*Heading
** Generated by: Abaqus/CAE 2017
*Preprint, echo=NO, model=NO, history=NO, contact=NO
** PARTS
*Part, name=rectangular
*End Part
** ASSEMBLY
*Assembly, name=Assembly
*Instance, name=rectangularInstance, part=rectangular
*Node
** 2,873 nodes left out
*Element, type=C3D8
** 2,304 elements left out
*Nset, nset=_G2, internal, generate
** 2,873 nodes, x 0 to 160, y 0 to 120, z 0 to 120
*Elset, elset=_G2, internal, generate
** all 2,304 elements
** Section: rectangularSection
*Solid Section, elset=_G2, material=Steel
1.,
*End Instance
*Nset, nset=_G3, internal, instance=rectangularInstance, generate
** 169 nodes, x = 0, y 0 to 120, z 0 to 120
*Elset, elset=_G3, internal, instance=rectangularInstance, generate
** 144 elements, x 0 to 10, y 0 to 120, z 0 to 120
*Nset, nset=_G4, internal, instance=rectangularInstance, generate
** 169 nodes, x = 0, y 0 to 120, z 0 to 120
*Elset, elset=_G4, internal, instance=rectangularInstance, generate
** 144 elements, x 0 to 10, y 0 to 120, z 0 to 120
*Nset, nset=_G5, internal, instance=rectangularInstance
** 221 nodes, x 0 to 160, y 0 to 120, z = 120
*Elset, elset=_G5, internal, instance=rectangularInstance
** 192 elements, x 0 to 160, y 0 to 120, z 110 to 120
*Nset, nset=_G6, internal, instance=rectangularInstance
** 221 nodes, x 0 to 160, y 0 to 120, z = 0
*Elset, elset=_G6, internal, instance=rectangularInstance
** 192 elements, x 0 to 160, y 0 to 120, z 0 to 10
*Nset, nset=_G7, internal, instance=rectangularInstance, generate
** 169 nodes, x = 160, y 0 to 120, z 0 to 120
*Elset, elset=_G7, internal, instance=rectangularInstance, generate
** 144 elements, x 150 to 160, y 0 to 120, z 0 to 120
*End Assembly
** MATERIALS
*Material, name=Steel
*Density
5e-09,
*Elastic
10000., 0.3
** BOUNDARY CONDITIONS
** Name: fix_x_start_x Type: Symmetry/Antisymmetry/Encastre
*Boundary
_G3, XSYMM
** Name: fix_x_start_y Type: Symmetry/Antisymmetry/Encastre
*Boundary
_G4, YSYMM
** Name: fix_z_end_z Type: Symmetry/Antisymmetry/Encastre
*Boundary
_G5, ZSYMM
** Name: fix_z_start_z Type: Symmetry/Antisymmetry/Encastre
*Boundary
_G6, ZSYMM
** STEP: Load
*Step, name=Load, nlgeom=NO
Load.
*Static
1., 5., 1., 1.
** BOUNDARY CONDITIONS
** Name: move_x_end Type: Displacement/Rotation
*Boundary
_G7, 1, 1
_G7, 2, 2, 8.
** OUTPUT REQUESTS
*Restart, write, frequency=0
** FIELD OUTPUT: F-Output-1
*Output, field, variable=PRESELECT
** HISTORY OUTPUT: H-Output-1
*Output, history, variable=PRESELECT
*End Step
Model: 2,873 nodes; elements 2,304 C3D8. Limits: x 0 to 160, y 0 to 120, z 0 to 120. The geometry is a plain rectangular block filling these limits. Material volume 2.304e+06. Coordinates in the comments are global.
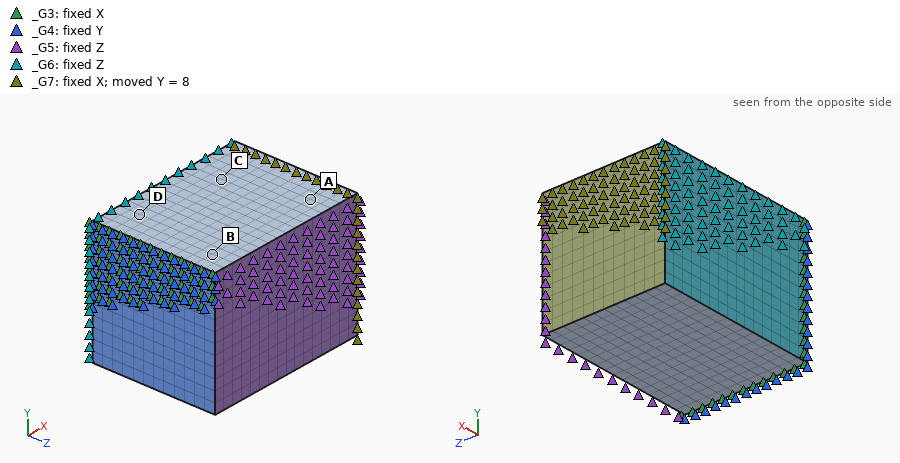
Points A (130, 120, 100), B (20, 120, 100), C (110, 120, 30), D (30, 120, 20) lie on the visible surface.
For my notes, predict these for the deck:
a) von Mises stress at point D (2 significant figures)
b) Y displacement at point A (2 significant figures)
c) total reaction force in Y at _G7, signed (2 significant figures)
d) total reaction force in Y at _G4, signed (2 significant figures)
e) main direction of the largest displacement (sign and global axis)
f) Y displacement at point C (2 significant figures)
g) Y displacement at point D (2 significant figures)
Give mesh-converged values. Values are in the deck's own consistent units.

250
6.6
1.6e+06
-1.6e+06
+Y
5.6
1.4
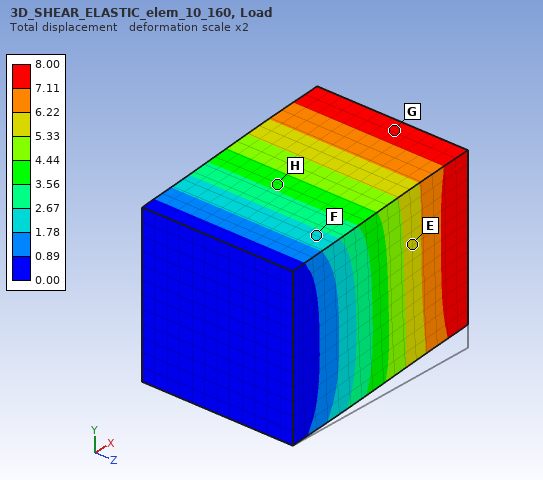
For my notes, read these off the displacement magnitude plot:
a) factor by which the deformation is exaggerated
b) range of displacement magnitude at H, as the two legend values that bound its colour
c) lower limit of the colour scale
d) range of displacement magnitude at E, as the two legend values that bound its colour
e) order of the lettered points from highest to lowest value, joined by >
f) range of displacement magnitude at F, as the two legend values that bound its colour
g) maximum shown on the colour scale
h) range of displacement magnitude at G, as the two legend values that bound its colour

2
3.56 to 4.44
0.00
5.33 to 6.22
G > E > H > F
1.78 to 2.67
8.00
7.11 to 8.00
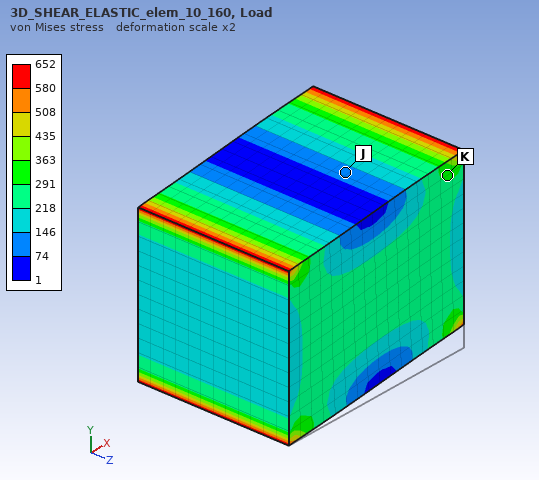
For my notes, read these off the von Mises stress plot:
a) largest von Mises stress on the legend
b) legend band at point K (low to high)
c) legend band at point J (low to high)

652
291 to 363
74 to 146
